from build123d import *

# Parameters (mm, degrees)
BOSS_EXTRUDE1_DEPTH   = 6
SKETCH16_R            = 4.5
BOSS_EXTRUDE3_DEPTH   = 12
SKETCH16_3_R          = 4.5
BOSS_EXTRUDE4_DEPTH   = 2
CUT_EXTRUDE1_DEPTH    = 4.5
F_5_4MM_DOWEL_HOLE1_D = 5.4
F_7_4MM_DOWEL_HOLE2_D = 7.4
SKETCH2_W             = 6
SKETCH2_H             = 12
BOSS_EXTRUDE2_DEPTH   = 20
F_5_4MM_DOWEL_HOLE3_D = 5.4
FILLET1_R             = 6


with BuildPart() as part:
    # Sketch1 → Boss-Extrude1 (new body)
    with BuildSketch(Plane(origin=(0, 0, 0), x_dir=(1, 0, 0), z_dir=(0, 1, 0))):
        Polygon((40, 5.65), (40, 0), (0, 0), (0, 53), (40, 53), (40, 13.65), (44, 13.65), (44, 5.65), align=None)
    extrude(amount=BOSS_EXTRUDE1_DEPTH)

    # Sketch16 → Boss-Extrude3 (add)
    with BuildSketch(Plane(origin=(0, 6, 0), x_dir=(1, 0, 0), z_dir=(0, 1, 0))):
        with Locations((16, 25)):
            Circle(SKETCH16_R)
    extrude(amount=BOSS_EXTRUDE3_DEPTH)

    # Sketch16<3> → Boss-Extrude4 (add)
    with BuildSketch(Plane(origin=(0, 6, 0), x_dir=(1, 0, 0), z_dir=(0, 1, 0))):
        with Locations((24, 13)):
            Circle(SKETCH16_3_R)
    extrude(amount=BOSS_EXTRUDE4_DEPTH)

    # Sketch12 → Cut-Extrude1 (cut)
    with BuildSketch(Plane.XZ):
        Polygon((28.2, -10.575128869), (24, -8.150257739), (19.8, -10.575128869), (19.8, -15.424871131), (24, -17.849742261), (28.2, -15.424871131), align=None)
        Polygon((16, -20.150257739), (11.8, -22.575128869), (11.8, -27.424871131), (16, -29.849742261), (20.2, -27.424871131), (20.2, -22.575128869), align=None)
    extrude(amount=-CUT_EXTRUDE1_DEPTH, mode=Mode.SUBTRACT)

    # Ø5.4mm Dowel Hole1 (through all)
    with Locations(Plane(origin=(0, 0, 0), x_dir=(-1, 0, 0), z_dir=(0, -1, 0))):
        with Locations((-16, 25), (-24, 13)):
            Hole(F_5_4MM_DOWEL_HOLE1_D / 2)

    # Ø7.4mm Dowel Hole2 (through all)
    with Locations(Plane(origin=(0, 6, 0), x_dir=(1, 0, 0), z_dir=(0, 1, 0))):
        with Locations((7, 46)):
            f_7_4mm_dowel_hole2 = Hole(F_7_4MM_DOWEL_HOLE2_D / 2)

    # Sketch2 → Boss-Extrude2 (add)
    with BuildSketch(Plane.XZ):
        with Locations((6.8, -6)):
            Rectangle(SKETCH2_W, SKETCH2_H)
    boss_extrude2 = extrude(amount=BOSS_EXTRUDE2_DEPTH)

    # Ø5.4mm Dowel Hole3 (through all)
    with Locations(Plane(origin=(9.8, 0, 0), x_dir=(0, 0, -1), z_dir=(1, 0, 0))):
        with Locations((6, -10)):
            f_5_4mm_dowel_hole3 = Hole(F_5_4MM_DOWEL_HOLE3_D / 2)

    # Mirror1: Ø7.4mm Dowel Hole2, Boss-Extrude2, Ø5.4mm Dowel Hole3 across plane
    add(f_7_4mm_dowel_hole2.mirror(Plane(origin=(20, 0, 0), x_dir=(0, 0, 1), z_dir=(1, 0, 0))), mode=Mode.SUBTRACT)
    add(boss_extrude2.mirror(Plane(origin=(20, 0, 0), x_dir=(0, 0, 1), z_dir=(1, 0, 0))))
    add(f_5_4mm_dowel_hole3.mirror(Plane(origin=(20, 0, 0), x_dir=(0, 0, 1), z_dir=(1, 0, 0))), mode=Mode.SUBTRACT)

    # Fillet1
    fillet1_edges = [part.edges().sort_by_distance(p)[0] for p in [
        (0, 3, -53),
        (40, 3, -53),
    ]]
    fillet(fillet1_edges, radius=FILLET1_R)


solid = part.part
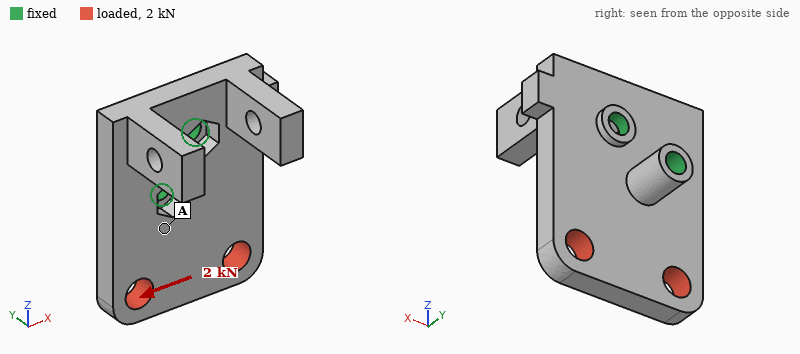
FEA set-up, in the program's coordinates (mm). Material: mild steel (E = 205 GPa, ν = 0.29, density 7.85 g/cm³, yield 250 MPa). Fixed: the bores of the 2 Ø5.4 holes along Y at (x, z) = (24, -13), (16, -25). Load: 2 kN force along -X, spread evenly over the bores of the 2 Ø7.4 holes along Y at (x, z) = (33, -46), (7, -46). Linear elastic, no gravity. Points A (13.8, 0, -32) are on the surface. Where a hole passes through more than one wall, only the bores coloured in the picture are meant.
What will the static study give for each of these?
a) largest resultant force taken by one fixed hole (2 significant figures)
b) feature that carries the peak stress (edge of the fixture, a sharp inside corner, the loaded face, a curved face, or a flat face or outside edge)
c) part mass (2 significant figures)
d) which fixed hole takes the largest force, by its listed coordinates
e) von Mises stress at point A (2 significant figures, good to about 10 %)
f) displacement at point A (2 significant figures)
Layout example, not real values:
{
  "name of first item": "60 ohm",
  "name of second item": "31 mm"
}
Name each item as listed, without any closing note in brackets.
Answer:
{
  "largest resultant force taken by one fixed hole": "3.7 kN",
  "feature that carries the peak stress": "edge of the fixture",
  "part mass": "120 g",
  "which fixed hole takes the largest force, by its listed coordinates": "(16, -25)",
  "von Mises stress at point A": "34 MPa",
  "displacement at point A": "8.0 µm"
}
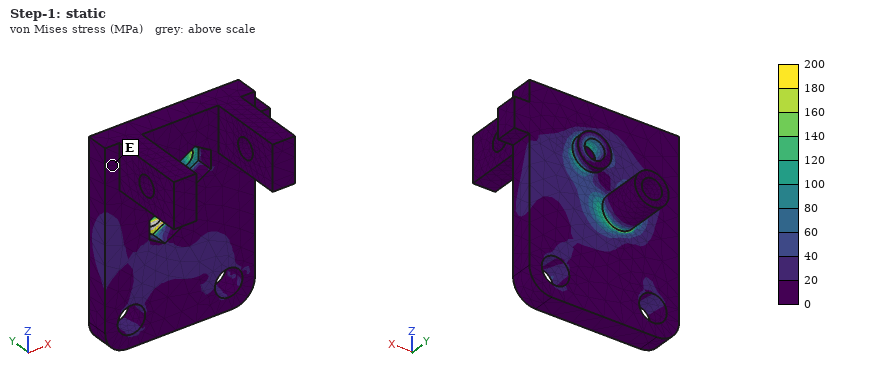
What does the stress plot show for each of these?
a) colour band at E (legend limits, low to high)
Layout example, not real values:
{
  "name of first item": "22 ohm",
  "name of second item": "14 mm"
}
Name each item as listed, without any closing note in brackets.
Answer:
{
  "colour band at E": "0 to 20 MPa"
}
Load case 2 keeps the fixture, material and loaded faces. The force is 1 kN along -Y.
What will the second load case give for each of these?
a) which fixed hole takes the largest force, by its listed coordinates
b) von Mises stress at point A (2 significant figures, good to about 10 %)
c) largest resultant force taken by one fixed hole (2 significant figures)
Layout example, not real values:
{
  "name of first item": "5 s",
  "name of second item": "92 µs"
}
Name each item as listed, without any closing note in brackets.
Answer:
{
  "which fixed hole takes the largest force, by its listed coordinates": "(16, -25)",
  "von Mises stress at point A": "75 MPa",
  "largest resultant force taken by one fixed hole": "1.9 kN"
}
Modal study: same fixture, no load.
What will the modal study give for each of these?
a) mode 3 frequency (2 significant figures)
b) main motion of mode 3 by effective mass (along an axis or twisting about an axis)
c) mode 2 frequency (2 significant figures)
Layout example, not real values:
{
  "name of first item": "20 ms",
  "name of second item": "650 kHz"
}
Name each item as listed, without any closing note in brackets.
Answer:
{
  "mode 3 frequency": "6000 Hz",
  "main motion of mode 3 by effective mass": "along Y",
  "mode 2 frequency": "5100 Hz"
}
